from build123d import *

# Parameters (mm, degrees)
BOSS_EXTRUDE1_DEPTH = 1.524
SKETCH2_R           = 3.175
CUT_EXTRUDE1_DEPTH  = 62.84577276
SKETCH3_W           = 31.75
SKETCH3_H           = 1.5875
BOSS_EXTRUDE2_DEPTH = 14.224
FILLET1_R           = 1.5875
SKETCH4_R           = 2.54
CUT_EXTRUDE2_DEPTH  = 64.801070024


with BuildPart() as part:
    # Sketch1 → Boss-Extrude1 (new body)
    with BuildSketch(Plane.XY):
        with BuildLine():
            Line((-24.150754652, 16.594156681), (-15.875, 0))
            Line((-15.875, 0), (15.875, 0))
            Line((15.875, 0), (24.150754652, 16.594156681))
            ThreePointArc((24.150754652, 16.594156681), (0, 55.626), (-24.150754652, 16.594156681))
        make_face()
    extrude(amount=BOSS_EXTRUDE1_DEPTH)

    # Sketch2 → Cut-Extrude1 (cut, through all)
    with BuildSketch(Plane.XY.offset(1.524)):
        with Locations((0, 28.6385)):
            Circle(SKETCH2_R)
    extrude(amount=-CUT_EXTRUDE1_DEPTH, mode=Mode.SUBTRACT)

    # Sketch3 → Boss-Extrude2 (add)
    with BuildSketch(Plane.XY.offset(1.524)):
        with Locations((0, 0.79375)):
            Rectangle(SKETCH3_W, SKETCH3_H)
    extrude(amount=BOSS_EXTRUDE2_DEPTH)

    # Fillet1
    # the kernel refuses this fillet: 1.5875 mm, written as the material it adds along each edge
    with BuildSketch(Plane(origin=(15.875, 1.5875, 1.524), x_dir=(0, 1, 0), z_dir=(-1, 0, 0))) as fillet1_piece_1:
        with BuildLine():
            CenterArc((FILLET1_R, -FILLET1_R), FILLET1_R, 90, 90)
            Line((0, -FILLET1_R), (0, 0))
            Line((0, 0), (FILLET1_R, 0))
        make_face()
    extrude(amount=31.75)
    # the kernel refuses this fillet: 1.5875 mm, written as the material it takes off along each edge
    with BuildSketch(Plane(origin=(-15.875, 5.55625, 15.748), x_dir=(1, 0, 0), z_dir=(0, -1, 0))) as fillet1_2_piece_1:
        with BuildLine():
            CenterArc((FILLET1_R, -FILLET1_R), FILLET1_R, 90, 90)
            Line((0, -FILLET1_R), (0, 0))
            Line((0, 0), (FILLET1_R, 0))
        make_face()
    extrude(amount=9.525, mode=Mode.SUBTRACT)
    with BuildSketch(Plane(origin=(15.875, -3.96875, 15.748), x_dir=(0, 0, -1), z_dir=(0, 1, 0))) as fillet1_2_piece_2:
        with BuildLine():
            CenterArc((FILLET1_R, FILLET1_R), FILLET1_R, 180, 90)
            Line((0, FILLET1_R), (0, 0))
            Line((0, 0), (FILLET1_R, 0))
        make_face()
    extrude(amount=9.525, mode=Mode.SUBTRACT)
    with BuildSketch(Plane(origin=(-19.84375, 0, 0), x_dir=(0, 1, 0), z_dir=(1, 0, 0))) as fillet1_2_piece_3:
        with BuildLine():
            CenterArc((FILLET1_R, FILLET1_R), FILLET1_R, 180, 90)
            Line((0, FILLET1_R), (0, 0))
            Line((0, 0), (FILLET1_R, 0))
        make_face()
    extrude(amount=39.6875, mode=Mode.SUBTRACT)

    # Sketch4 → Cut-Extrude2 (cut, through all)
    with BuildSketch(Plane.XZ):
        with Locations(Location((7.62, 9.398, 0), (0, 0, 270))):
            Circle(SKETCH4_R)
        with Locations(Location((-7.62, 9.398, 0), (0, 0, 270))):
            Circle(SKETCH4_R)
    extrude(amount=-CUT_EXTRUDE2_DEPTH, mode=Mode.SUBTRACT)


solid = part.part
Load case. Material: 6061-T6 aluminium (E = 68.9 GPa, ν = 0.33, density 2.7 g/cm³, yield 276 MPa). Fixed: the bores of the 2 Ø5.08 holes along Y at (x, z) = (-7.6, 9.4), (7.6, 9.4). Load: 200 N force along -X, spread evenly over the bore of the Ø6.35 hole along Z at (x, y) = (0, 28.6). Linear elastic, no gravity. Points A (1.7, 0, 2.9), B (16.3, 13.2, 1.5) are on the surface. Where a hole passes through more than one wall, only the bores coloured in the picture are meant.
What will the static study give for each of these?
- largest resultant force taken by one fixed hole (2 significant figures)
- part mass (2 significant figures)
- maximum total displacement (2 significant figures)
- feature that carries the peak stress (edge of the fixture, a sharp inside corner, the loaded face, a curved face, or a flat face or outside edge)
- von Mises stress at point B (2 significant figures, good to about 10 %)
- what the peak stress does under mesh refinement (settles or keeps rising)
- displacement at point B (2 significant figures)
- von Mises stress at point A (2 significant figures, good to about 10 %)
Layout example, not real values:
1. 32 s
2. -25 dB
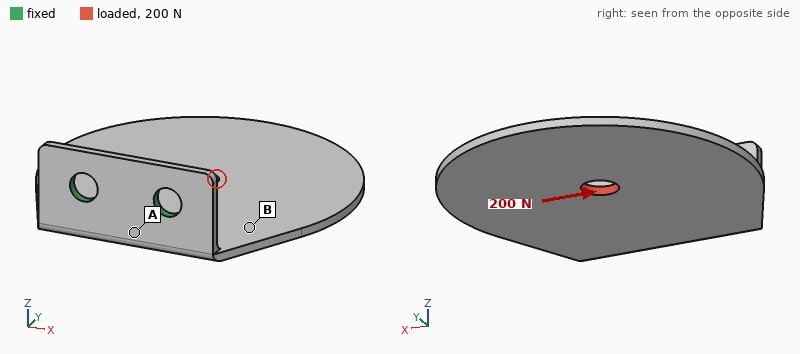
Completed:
1. 320 N
2. 12 g
3. 0.38 mm
4. edge of the fixture
5. 28 MPa
6. keeps rising
7. 0.17 mm
8. 74 MPa
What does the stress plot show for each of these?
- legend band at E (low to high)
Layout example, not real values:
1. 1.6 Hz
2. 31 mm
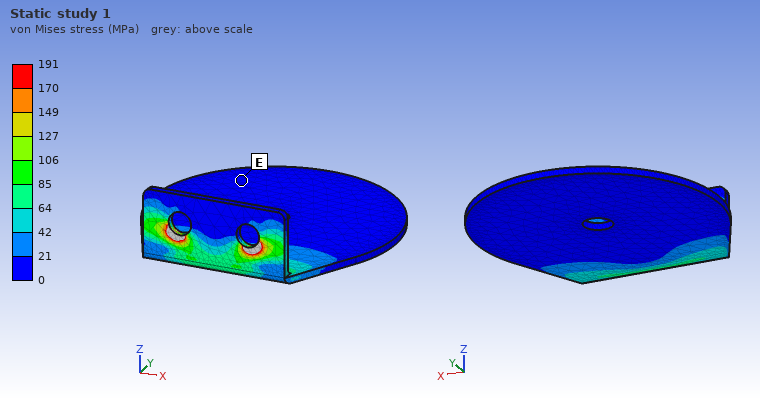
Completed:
1. 0 to 21 MPa
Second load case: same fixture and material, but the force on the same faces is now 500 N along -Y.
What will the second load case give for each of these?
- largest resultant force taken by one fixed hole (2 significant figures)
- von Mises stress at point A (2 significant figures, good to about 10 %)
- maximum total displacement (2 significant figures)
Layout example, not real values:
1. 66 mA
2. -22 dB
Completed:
1. 250 N
2. 76 MPa
3. 0.89 mm
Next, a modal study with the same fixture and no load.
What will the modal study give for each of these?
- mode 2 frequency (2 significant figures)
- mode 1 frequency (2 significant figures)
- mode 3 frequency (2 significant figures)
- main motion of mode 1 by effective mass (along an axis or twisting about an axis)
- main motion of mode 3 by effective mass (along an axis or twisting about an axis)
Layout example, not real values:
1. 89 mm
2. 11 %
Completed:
1. 1000 Hz
2. 370 Hz
3. 1500 Hz
4. along Z
5. along X
